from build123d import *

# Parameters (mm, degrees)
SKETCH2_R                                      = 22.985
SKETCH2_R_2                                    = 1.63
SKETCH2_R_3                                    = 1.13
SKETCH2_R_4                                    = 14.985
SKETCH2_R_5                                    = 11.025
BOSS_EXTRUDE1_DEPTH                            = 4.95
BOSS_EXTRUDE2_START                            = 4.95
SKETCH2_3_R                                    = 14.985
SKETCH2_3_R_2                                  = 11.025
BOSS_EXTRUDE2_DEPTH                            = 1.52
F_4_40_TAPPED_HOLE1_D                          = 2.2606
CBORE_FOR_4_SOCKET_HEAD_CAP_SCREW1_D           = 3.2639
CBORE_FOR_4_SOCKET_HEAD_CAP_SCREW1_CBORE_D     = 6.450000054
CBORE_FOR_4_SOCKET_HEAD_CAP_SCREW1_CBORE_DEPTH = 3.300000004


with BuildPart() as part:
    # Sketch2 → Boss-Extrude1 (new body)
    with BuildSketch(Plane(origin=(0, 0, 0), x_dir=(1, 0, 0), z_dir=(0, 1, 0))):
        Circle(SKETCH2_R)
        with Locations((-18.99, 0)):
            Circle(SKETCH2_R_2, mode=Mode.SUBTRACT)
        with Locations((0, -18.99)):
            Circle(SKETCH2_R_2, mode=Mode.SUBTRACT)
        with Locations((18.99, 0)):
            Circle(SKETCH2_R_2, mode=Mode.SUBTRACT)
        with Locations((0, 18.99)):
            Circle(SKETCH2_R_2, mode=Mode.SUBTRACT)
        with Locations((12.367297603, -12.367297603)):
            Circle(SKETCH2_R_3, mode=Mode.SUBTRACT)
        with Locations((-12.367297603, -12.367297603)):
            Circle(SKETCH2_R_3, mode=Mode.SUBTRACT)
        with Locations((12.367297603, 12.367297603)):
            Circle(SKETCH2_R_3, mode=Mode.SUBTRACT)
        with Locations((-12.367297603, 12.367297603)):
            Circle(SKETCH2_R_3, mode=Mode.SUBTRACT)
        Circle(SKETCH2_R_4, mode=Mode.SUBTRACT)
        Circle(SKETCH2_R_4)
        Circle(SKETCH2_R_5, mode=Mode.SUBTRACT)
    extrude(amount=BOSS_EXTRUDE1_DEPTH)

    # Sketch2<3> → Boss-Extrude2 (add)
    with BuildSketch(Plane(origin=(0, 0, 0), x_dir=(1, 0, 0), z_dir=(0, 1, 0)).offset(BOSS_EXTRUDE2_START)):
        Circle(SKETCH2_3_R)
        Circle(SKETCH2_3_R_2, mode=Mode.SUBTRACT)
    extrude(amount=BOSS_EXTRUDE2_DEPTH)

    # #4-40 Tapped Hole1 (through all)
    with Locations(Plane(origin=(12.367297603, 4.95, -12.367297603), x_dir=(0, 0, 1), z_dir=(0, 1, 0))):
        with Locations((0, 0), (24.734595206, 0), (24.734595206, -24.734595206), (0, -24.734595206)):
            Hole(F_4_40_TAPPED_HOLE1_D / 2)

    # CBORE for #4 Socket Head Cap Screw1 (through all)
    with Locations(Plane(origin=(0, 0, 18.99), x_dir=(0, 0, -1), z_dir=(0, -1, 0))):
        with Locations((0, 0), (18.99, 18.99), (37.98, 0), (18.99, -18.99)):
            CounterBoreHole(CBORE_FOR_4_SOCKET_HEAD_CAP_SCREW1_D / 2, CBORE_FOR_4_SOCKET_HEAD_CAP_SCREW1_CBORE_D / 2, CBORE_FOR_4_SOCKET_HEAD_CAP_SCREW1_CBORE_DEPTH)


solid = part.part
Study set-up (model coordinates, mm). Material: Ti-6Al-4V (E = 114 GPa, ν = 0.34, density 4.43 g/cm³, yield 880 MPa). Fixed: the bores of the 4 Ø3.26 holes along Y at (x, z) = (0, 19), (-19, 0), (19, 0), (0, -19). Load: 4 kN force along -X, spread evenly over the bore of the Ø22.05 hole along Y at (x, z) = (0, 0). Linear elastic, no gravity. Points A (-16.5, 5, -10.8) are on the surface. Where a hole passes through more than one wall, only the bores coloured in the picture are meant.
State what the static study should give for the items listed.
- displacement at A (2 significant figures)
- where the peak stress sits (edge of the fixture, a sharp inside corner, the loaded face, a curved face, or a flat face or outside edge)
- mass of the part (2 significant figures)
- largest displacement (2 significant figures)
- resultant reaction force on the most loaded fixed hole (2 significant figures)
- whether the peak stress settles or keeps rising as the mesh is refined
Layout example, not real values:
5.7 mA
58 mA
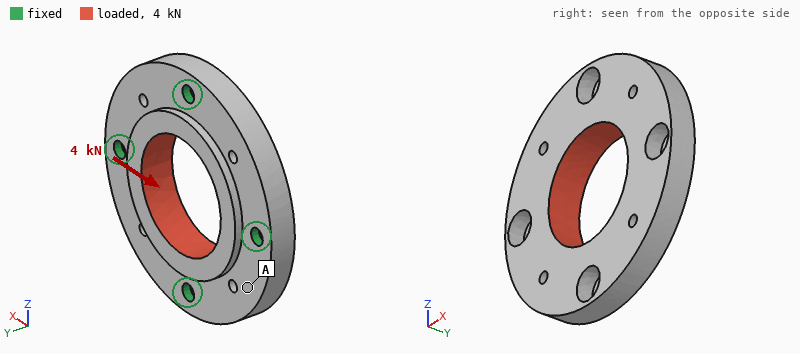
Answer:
3.0 µm
edge of the fixture
28 g
4.2 µm
1.0 kN
keeps rising
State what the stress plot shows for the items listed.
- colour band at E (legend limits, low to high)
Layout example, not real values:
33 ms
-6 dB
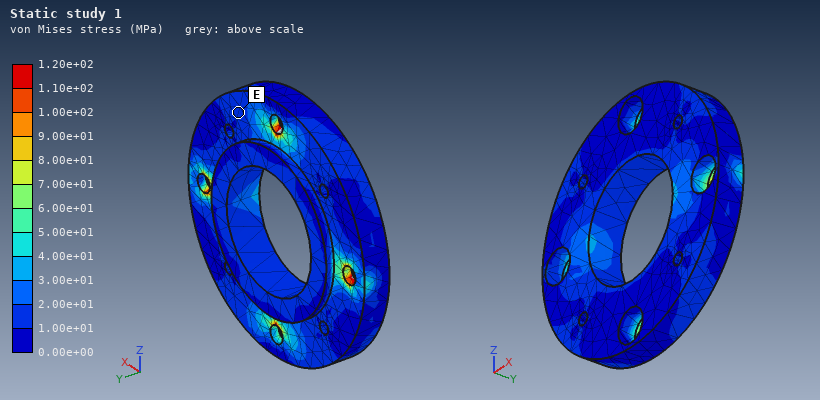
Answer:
1.00e+01 to 2.00e+01 MPa
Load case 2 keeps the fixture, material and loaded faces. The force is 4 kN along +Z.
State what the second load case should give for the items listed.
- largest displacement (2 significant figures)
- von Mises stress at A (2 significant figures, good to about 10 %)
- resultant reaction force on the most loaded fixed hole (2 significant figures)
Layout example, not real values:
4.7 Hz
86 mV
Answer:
4.2 µm
13 MPa
1.0 kN
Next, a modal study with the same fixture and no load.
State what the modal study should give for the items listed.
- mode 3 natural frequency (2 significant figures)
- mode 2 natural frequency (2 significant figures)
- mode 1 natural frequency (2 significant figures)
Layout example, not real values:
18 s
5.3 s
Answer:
18 kHz
18 kHz
15 kHz
